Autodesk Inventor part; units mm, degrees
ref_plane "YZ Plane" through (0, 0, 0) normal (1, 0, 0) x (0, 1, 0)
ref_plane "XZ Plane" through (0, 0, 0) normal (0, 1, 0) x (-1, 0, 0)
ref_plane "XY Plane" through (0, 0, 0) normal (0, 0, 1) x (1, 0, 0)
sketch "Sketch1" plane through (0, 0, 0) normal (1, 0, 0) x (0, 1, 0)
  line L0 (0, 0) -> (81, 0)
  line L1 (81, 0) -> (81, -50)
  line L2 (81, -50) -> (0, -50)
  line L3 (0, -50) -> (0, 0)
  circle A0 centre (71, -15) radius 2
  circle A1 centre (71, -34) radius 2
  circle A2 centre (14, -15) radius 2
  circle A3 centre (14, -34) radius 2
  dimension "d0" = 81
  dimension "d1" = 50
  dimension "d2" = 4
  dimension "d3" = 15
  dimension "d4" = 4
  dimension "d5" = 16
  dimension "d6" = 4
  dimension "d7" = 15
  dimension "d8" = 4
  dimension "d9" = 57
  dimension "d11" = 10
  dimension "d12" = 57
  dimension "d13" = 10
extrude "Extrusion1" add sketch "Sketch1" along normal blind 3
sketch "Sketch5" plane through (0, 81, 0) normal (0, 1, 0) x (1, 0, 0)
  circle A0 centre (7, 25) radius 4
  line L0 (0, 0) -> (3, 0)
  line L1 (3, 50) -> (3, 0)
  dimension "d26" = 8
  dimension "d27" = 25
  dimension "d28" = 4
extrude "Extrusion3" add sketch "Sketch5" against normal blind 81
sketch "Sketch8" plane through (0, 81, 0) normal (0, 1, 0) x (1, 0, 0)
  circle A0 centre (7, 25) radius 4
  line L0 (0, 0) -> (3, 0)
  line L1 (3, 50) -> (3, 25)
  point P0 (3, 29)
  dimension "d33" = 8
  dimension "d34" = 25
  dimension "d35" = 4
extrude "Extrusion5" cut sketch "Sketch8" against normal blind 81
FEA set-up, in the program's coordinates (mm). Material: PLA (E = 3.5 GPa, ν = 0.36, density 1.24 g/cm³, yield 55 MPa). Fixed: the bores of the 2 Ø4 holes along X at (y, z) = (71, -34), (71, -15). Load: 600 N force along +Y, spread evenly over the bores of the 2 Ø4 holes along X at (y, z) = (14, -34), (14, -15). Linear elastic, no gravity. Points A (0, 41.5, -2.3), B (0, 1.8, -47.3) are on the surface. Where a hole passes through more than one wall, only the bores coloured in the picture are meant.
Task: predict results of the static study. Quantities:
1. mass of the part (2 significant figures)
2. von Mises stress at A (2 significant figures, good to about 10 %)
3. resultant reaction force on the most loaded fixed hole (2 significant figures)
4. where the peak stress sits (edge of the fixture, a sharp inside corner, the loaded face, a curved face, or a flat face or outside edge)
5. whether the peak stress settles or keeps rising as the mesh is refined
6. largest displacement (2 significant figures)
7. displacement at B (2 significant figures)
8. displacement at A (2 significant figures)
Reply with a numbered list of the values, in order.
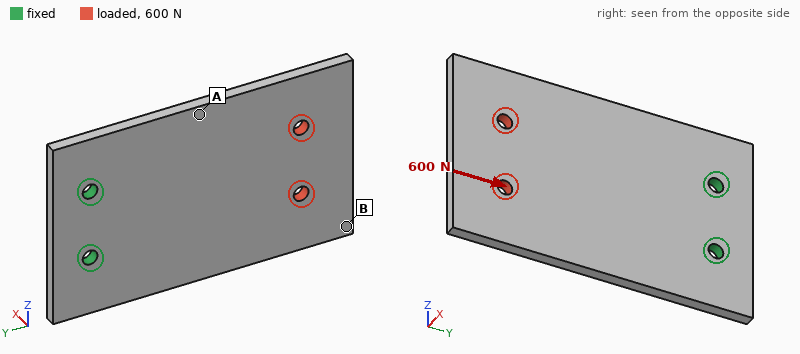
1. 15 g
2. 3.5 MPa
3. 300 N
4. edge of the fixture
5. keeps rising
6. 93 µm
7. 65 µm
8. 47 µm
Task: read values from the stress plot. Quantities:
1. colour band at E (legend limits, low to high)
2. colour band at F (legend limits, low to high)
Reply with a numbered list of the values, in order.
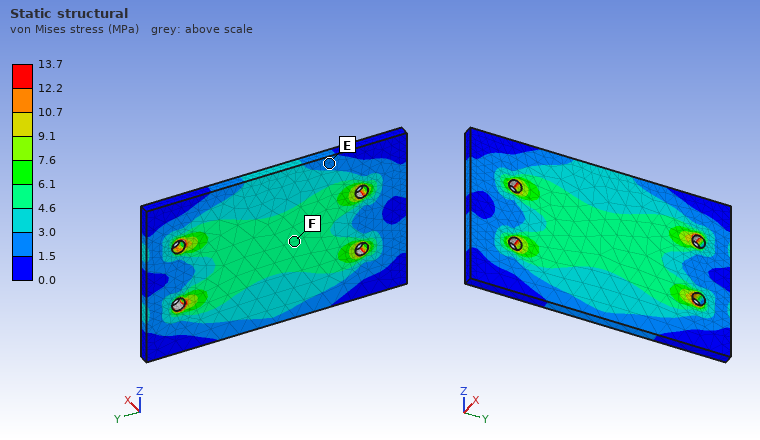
1. 1.5 to 3.0 MPa
2. 4.6 to 6.1 MPa
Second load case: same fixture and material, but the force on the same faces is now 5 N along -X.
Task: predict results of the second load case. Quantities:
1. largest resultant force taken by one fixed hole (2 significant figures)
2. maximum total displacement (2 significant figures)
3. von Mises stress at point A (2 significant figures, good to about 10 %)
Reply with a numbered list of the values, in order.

1. 2.5 N
2. 1.1 mm
3. 1.9 MPa
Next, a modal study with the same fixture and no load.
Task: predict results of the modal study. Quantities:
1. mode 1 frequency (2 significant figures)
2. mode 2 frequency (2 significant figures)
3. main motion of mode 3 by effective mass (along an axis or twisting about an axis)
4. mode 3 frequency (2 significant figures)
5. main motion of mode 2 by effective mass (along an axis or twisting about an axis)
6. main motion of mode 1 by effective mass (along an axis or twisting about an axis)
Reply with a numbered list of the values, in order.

1. 160 Hz
2. 490 Hz
3. along X
4. 990 Hz
5. twisting about Y
6. along X
